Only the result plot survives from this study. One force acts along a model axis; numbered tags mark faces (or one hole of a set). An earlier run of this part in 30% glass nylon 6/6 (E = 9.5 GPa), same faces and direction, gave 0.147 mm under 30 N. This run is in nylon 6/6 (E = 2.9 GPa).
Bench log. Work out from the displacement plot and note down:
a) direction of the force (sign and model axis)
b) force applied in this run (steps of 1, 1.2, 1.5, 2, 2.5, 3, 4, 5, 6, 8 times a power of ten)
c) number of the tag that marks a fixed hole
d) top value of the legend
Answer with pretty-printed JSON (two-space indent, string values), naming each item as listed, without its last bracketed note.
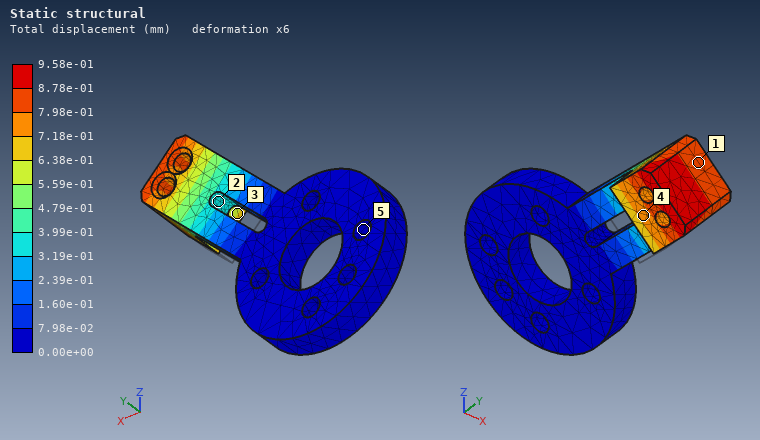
{
  "direction of the force": "+Y",
  "force applied in this run": "60 N",
  "number of the tag that marks a fixed hole": "5",
  "top value of the legend": "9.58e-01 mm"
}
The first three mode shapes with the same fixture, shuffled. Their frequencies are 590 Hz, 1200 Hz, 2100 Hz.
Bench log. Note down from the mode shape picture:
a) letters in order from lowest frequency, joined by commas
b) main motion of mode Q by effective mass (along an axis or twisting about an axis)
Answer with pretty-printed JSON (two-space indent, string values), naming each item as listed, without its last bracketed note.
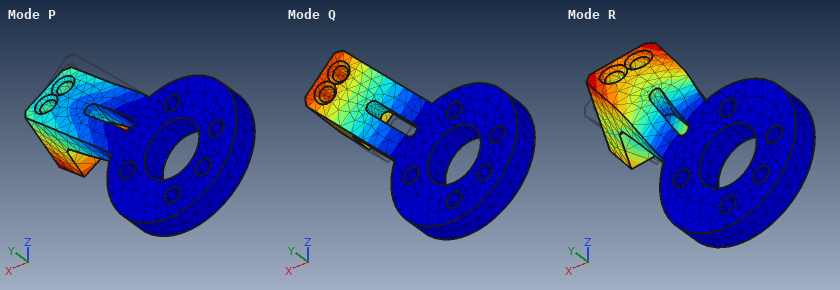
{
  "letters in order from lowest frequency, joined by commas": "Q, P, R",
  "main motion of mode Q by effective mass": "along Y"
}
